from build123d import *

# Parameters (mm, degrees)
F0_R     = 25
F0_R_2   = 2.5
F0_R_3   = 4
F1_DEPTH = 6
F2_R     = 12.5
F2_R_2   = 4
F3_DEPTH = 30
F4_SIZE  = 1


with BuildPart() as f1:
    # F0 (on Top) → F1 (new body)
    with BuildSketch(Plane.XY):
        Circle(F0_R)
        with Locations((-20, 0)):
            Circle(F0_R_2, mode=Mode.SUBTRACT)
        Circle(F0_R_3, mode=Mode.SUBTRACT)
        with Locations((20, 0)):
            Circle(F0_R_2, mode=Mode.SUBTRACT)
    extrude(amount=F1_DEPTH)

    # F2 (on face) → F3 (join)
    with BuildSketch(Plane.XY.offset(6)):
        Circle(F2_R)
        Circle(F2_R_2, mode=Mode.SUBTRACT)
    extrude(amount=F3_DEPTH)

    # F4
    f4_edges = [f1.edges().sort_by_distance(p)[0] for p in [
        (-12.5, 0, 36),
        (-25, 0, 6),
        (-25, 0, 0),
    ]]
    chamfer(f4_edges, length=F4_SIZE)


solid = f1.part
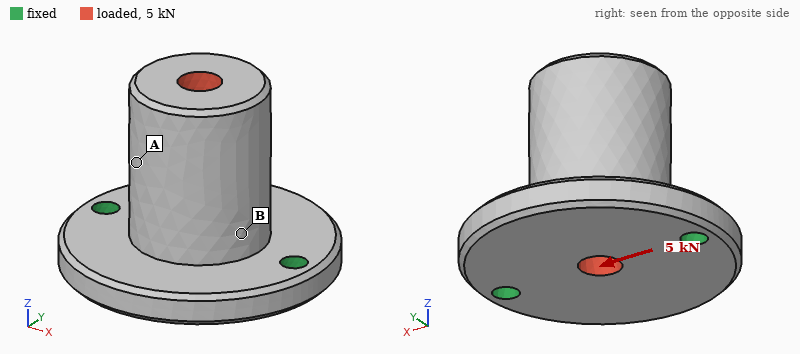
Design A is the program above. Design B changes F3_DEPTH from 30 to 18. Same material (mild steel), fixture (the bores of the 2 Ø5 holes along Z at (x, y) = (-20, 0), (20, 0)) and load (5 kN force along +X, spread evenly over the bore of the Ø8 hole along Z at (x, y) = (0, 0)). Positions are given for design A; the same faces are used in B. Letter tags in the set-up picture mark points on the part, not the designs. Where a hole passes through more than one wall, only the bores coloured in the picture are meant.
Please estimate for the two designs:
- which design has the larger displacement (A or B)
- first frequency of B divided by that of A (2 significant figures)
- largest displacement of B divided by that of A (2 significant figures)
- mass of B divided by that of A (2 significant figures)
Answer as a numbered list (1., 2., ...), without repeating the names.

1. A
2. 1.5
3. 0.41
4. 0.78
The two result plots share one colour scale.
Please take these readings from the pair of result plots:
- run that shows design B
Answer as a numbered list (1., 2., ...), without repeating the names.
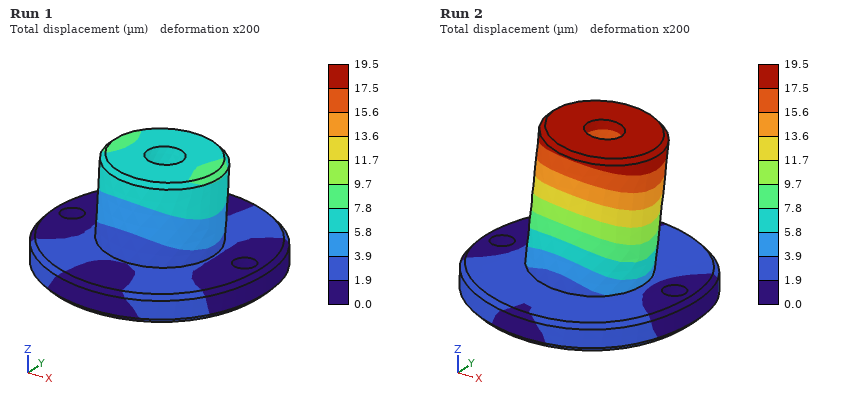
1. Run 1
